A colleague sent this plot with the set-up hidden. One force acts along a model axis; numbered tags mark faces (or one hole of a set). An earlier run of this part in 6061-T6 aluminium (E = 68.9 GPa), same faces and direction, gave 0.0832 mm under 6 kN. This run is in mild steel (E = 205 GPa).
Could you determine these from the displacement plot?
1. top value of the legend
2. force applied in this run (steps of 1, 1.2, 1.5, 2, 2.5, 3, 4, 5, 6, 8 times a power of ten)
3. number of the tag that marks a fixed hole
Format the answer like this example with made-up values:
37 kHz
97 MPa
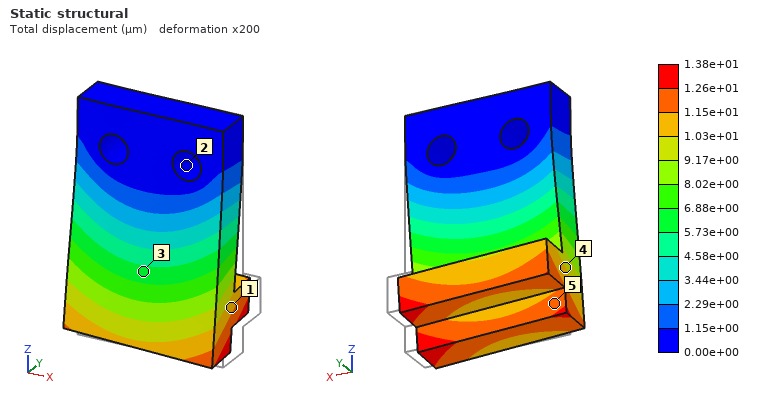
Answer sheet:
1.38e+01 µm
3 kN
2
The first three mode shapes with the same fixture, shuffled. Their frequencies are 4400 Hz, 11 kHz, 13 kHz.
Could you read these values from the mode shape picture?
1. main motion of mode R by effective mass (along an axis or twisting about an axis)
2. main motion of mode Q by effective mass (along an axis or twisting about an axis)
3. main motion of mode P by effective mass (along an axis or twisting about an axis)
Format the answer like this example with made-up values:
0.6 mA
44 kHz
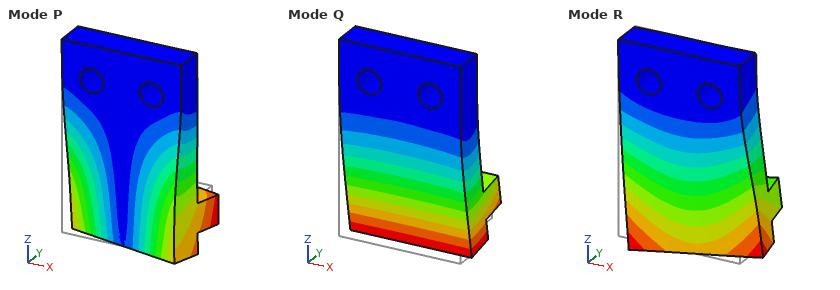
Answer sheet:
along X
along Y
along X
